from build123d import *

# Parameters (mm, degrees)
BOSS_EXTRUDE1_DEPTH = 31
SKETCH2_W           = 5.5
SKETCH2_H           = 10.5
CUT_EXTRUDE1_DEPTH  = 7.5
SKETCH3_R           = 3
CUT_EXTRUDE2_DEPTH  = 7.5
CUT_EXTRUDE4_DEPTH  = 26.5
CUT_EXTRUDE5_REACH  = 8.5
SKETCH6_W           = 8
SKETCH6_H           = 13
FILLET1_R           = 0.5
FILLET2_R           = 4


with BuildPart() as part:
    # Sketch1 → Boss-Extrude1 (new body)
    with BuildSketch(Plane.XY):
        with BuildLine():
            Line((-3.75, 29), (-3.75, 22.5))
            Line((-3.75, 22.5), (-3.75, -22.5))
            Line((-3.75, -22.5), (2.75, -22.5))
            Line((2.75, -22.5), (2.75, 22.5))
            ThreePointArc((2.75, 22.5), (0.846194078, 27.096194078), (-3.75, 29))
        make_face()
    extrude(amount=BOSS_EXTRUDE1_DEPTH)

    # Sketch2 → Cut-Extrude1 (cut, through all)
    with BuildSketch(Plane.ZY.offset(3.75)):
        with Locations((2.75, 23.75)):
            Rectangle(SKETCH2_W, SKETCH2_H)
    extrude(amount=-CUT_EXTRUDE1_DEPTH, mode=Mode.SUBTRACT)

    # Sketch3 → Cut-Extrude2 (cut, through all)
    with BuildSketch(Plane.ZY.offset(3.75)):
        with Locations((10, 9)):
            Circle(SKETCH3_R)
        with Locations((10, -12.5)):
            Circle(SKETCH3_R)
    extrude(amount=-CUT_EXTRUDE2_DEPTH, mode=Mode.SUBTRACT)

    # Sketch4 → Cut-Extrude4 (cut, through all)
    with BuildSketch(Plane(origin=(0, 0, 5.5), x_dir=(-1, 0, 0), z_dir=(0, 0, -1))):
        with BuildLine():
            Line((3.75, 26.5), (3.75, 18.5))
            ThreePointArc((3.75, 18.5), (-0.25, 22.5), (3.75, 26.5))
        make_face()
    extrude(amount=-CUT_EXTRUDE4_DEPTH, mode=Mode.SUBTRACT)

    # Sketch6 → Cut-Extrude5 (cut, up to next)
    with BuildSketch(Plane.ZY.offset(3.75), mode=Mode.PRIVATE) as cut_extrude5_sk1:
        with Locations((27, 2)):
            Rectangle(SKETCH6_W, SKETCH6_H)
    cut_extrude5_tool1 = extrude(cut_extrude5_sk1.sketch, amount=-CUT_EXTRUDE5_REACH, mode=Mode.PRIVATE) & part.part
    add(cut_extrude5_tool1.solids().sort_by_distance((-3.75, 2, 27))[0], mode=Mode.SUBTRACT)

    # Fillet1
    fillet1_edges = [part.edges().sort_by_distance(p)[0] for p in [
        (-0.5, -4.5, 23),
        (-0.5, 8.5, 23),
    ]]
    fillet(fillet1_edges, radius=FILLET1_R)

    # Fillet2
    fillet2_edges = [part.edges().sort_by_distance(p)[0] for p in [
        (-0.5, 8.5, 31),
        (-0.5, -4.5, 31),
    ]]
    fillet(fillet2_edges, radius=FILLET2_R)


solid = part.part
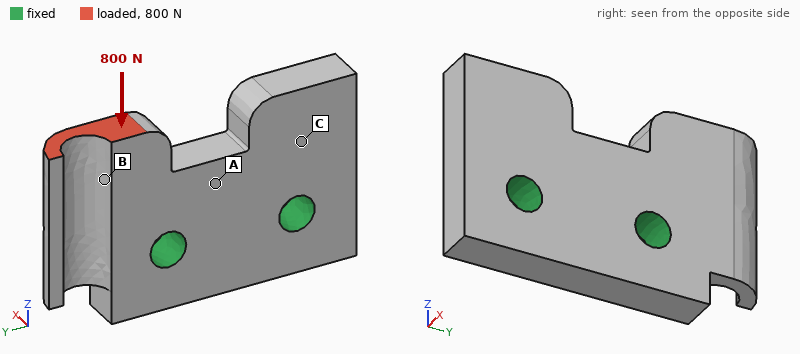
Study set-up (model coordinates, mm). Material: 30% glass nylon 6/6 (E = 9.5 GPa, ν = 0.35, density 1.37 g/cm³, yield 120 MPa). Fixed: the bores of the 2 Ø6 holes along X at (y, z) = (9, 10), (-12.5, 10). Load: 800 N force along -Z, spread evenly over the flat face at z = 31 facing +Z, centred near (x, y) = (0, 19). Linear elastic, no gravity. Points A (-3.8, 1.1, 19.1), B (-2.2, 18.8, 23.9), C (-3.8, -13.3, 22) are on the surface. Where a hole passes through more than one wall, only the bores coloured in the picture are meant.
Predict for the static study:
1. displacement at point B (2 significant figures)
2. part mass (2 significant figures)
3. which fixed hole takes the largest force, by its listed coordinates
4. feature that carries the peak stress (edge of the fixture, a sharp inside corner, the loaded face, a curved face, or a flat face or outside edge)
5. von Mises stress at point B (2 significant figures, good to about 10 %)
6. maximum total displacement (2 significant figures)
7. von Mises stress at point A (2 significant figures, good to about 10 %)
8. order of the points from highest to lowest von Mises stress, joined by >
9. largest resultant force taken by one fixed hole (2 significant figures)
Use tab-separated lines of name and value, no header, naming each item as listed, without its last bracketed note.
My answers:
displacement at point B	0.049 mm
part mass	11 g
which fixed hole takes the largest force, by its listed coordinates	(9, 10)
feature that carries the peak stress	a curved face
von Mises stress at point B	15 MPa
maximum total displacement	0.11 mm
von Mises stress at point A	6.0 MPa
order of the points from highest to lowest von Mises stress, joined by >	B > A > C
largest resultant force taken by one fixed hole	1.0 kN
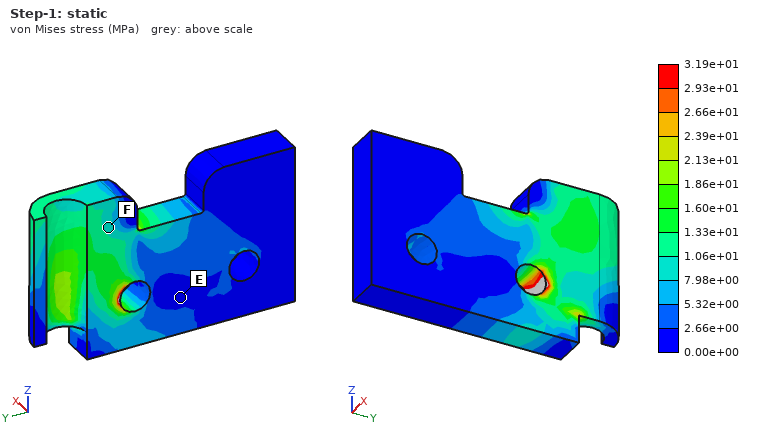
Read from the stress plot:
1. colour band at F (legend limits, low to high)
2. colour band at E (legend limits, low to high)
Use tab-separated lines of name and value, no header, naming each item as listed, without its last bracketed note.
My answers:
colour band at F	7.98e+00 to 1.06e+01 MPa
colour band at E	0.00e+00 to 2.66e+00 MPa
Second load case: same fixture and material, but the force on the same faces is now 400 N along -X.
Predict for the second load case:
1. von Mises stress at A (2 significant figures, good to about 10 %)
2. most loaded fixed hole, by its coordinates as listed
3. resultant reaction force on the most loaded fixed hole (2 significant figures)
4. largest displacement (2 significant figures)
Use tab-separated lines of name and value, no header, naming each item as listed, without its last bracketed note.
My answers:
von Mises stress at A	21 MPa
most loaded fixed hole, by its coordinates as listed	(9, 10)
resultant reaction force on the most loaded fixed hole	470 N
largest displacement	0.67 mm
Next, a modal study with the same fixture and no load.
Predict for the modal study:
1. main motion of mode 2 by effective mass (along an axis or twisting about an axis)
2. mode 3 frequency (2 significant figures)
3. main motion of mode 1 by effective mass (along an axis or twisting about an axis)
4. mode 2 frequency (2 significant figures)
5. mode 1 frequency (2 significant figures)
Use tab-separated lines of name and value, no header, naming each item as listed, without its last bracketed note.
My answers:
main motion of mode 2 by effective mass	along X
mode 3 frequency	8400 Hz
main motion of mode 1 by effective mass	along X
mode 2 frequency	7200 Hz
mode 1 frequency	5400 Hz
